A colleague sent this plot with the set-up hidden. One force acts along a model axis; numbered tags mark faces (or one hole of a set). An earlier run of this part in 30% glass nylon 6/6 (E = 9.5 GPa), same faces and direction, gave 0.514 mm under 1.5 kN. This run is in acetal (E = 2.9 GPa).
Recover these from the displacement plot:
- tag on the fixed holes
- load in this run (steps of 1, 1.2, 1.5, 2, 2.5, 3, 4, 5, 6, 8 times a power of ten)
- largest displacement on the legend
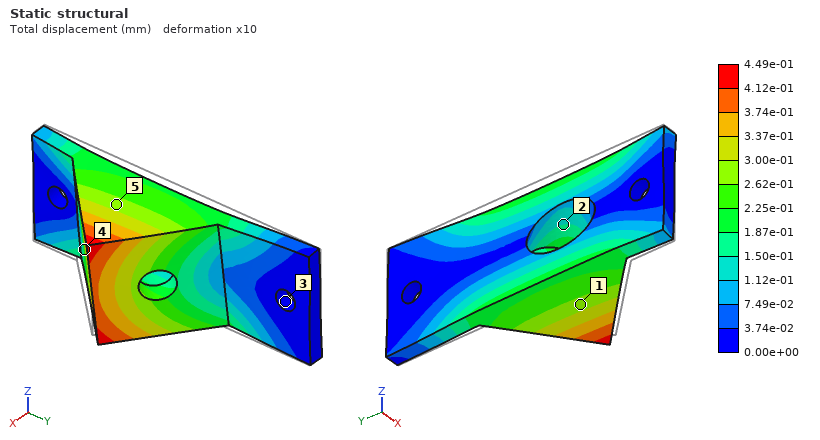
3
400 N
4.49e-01 mm
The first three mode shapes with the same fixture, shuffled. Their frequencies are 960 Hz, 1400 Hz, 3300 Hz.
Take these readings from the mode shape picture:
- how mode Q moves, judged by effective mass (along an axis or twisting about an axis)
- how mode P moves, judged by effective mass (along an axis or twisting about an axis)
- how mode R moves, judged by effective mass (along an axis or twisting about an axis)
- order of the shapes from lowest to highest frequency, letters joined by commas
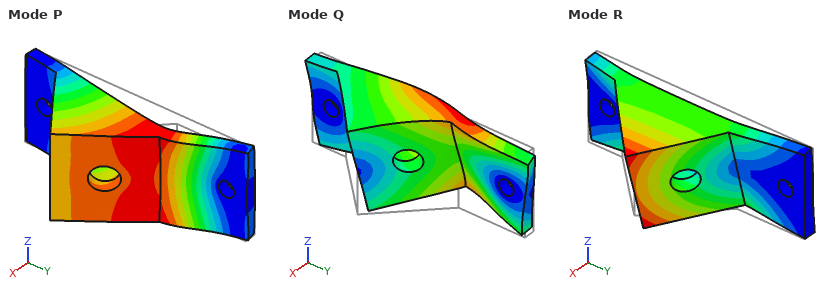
along Z
along X
along Z
R, P, Q
